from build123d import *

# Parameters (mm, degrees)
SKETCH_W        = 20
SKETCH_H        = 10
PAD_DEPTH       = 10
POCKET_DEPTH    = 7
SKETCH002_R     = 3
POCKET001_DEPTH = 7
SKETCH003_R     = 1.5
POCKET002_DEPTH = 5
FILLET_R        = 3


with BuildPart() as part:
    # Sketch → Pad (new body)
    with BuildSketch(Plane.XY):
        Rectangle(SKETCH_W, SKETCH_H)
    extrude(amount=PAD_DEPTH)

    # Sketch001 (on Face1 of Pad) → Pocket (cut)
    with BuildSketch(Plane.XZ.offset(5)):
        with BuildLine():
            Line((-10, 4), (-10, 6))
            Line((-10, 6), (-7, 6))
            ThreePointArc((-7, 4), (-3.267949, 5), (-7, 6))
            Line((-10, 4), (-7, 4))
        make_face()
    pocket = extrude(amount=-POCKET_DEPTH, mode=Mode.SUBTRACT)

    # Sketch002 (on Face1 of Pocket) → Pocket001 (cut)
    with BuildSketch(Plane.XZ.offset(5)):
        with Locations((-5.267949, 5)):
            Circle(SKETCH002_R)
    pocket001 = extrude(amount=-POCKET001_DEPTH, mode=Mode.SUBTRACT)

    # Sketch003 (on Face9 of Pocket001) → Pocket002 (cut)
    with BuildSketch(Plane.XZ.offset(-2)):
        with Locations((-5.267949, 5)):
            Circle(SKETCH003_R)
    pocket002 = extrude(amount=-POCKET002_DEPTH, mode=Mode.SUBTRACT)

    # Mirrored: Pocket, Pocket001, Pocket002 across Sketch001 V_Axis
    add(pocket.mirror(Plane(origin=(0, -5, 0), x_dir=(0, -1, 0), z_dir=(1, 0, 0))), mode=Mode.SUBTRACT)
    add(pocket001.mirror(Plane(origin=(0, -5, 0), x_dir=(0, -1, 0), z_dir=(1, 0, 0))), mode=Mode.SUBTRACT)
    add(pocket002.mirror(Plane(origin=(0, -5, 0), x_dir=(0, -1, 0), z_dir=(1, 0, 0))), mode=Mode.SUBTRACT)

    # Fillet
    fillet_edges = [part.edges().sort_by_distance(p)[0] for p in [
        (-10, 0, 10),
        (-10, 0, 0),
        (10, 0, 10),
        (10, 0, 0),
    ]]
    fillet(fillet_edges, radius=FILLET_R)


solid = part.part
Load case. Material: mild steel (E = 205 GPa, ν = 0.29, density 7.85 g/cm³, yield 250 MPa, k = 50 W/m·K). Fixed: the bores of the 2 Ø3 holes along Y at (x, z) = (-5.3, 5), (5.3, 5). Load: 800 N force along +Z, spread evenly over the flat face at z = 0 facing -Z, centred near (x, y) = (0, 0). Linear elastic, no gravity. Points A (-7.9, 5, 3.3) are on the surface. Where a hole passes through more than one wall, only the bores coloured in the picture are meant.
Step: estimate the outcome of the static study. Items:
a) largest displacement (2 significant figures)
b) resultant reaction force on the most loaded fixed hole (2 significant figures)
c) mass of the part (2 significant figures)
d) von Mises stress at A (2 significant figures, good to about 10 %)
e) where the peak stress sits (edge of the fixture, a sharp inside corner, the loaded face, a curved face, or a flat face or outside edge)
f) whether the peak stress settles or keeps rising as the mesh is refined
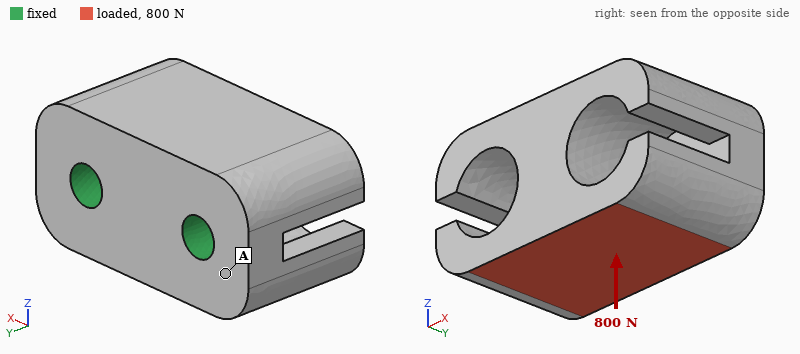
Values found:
4.6 µm
400 N
11 g
20 MPa
edge of the fixture
keeps rising
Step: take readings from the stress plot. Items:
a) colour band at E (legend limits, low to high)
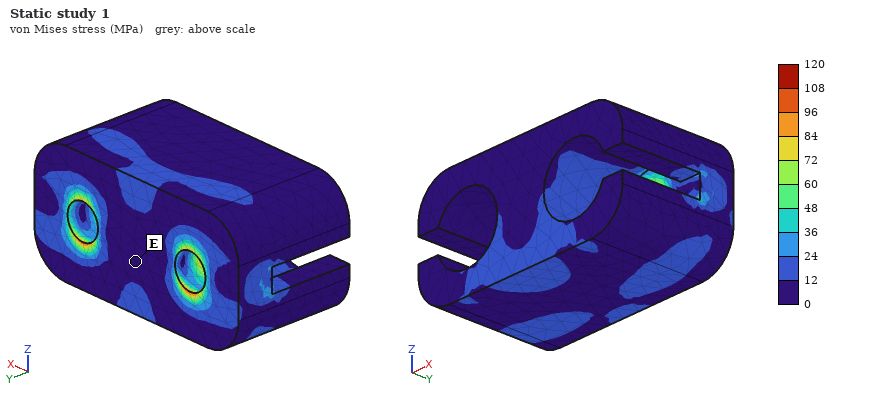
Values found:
0 to 12 MPa
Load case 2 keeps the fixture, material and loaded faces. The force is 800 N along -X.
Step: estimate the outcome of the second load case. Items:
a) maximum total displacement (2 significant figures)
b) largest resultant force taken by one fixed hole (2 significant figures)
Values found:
2.0 µm
540 N
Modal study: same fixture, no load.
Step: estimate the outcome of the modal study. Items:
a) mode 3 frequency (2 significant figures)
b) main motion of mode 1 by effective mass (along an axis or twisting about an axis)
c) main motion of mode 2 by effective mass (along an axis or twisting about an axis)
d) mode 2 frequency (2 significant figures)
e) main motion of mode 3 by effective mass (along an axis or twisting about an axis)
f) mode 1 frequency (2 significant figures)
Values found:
45 kHz
along Z
along X
41 kHz
twisting about Y
26 kHz
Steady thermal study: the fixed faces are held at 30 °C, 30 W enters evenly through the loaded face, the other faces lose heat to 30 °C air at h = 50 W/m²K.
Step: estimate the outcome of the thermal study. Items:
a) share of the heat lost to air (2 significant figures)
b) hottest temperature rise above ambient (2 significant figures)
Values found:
3.3 %
51 K
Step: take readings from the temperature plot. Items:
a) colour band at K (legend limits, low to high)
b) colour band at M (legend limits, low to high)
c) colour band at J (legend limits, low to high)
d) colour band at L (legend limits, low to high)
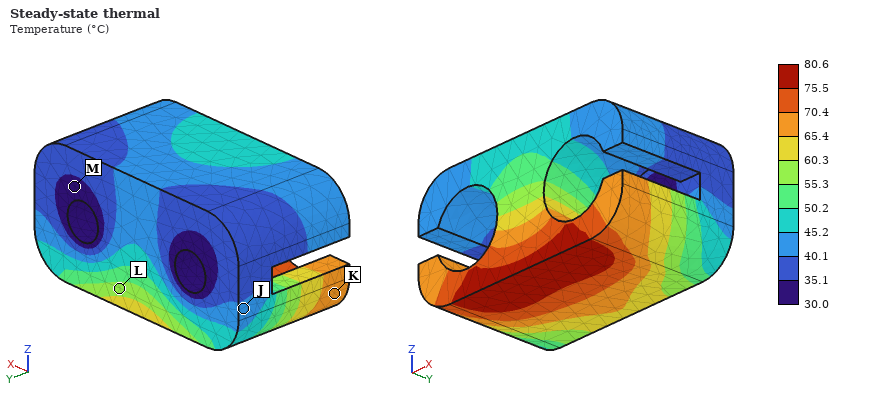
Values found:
65.4 to 70.4 °C
30.0 to 35.1 °C
40.1 to 45.2 °C
55.3 to 60.3 °C
